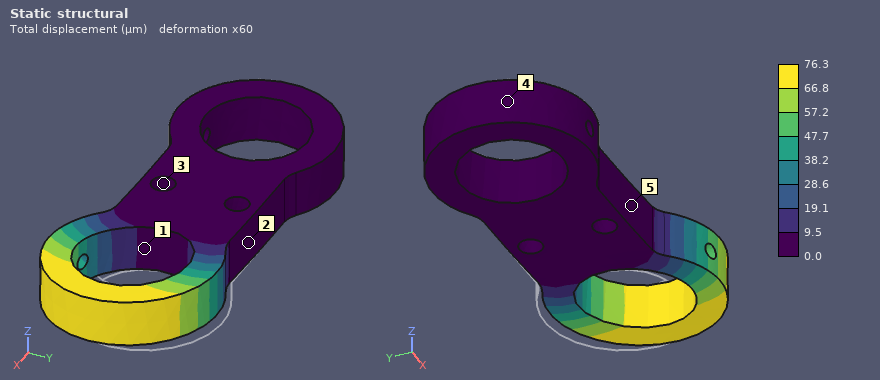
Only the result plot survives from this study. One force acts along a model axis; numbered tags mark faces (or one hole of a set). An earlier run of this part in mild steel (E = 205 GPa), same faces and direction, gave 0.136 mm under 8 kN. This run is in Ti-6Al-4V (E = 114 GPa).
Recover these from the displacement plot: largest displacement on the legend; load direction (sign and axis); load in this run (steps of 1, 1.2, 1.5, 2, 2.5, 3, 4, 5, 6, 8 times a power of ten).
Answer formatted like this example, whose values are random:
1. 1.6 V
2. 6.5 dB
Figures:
1. 76.3 µm
2. -Y
3. 2.5 kN
